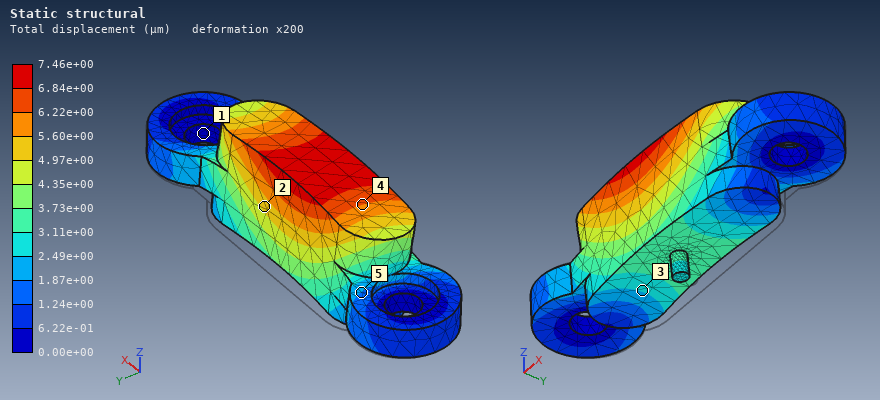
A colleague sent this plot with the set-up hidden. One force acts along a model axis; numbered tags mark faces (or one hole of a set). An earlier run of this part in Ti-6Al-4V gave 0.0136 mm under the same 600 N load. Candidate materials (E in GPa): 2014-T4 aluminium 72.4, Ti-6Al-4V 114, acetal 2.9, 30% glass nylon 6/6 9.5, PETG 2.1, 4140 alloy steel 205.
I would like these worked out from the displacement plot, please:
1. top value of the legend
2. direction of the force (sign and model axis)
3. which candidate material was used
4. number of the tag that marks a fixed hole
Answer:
7.46e+00 µm
-Y
4140 alloy steel
1
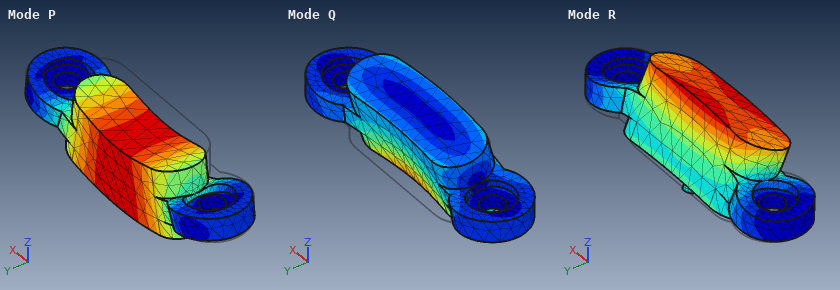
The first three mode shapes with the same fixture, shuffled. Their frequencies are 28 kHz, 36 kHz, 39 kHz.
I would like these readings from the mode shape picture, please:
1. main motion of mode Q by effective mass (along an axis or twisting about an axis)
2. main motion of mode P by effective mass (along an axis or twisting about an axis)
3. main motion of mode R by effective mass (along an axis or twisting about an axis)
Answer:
along Y
along Z
along Y
